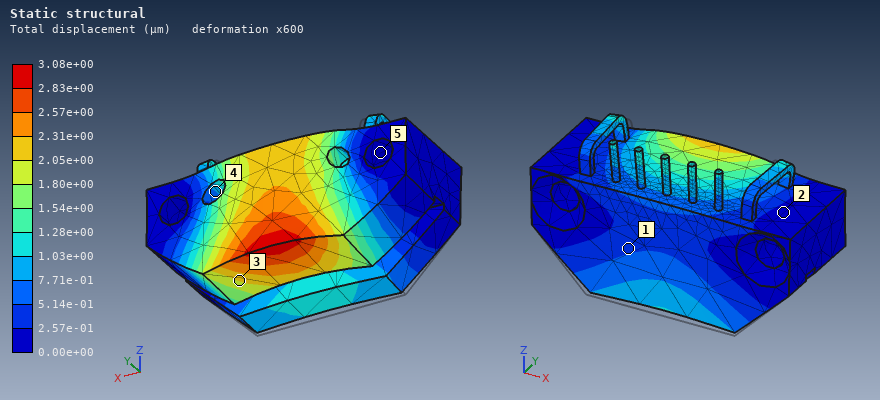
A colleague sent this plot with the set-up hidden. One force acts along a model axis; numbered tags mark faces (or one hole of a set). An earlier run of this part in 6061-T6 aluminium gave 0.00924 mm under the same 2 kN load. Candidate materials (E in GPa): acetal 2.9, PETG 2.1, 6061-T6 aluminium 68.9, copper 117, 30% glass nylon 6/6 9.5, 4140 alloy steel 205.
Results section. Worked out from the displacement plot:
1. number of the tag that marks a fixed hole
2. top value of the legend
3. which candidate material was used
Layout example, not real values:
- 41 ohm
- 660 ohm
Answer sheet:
- 5
- 3.08e+00 µm
- 4140 alloy steel
